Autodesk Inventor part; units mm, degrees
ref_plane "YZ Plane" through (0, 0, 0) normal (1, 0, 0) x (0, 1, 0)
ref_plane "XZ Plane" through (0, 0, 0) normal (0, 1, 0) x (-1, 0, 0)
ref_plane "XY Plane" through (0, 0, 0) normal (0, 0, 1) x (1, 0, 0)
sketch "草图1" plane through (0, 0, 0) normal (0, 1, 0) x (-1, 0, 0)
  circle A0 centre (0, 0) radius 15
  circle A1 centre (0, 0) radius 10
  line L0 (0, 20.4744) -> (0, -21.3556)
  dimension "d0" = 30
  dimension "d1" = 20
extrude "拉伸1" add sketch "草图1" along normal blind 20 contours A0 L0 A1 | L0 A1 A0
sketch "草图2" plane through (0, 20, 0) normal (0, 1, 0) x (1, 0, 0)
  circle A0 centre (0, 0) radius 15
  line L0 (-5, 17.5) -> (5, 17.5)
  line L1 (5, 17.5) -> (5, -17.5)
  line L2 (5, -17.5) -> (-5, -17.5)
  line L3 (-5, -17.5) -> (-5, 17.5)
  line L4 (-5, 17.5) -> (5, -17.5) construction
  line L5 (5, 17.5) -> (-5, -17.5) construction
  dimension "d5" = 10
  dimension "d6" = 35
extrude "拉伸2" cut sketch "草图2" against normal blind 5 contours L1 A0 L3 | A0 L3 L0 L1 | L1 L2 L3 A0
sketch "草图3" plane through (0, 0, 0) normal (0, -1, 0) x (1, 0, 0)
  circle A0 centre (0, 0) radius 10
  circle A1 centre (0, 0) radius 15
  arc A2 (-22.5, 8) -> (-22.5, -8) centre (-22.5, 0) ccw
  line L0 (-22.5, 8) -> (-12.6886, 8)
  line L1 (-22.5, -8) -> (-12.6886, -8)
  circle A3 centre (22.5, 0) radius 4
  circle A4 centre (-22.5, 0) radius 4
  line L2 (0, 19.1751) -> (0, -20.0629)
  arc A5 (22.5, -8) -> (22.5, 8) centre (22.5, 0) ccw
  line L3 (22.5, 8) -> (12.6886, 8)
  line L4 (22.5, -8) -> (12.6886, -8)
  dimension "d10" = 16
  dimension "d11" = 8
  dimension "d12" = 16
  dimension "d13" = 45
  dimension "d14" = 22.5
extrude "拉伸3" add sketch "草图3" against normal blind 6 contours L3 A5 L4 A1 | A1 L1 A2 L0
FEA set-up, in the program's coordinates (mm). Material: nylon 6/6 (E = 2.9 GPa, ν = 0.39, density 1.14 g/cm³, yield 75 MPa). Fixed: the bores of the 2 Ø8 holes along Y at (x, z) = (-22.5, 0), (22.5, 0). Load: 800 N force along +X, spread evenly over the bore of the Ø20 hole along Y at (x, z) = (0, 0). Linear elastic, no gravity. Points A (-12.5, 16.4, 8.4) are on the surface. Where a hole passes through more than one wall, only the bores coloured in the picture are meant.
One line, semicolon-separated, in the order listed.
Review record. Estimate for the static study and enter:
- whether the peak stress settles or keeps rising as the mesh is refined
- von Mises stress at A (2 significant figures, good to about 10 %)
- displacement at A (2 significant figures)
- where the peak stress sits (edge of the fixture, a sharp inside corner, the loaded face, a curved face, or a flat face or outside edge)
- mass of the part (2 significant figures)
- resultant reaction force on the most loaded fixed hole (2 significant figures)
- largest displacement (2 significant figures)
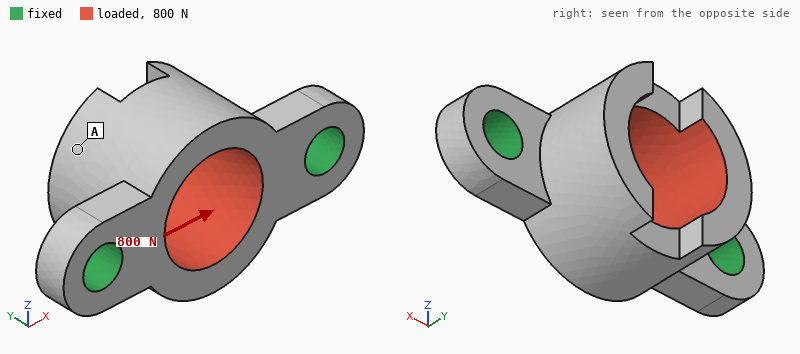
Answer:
keeps rising; 1.4 MPa; 52 µm; edge of the fixture; 11 g; 420 N; 64 µm
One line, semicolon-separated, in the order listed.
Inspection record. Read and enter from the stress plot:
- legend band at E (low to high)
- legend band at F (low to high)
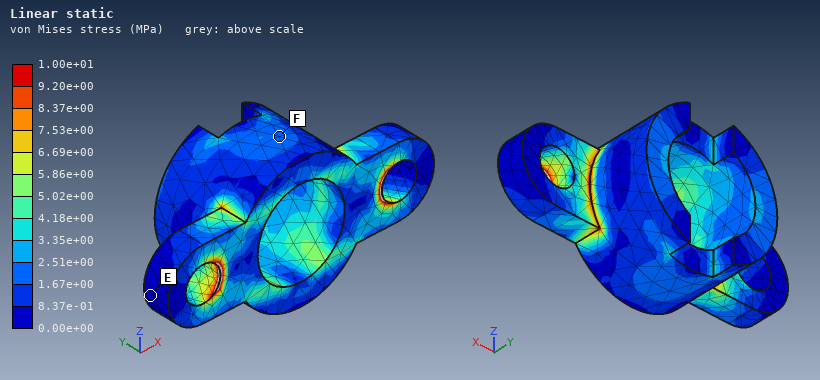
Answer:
0.00e+00 to 8.37e-01 MPa; 1.67e+00 to 2.51e+00 MPa
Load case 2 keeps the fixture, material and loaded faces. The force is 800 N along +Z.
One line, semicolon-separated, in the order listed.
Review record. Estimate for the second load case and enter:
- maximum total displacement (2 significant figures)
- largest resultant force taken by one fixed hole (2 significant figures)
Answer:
0.41 mm; 400 N
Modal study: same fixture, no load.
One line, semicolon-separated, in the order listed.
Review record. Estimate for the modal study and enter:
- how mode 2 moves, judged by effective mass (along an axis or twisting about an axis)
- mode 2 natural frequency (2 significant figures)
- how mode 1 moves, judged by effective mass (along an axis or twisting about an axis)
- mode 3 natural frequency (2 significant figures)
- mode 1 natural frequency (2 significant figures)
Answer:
along Y; 4400 Hz; along Z; 6200 Hz; 2500 Hz
